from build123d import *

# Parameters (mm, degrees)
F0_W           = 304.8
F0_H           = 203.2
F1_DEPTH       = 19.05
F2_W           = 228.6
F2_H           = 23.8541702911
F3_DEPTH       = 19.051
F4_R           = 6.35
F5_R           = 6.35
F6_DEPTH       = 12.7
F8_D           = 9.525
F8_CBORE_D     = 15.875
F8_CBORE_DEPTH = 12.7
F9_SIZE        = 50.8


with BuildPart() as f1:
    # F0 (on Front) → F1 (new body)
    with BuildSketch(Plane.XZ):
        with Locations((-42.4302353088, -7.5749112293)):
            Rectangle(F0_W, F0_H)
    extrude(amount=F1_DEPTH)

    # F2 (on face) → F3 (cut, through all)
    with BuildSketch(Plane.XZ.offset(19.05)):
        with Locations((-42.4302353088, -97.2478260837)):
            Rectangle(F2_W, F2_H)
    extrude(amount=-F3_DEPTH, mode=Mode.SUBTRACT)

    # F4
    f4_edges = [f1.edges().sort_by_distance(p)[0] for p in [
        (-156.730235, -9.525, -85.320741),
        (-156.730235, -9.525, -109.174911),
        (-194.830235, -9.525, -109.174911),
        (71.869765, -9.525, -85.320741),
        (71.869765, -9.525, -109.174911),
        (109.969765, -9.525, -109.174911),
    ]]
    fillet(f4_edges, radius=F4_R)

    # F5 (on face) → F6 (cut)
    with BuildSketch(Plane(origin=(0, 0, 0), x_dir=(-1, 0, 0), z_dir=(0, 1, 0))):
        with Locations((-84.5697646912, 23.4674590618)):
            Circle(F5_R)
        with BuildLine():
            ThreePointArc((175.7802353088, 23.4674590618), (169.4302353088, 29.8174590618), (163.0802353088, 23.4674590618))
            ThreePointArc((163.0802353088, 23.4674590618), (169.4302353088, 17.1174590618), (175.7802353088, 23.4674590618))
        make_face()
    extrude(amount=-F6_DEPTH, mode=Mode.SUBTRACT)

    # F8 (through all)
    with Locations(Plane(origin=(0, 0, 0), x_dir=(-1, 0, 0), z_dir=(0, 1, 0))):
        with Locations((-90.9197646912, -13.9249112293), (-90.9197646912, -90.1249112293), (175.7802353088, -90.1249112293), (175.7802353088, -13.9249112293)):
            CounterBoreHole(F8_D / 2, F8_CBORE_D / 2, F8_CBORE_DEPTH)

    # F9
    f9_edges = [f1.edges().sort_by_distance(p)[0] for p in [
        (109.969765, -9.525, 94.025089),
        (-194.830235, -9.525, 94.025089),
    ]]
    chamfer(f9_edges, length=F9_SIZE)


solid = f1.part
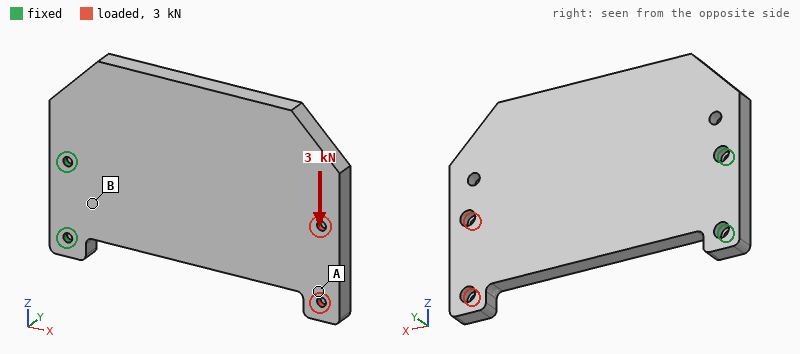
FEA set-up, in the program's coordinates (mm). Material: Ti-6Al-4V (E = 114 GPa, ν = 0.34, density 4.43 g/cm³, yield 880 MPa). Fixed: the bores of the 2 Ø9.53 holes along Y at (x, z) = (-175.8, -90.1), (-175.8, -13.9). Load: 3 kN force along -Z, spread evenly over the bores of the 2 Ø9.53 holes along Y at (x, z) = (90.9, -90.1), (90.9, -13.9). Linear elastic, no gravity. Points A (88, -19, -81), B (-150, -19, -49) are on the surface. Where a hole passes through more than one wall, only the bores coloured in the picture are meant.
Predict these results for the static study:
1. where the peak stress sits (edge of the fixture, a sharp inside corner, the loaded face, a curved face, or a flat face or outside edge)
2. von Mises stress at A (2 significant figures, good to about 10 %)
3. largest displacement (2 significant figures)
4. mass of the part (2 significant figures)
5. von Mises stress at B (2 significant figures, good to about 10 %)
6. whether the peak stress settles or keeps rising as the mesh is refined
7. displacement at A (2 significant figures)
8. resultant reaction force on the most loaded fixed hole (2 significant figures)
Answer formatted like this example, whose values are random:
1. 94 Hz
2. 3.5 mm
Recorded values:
1. edge of the fixture
2. 8.3 MPa
3. 0.18 mm
4. 4.5 kg
5. 17 MPa
6. keeps rising
7. 0.14 mm
8. 10 kN
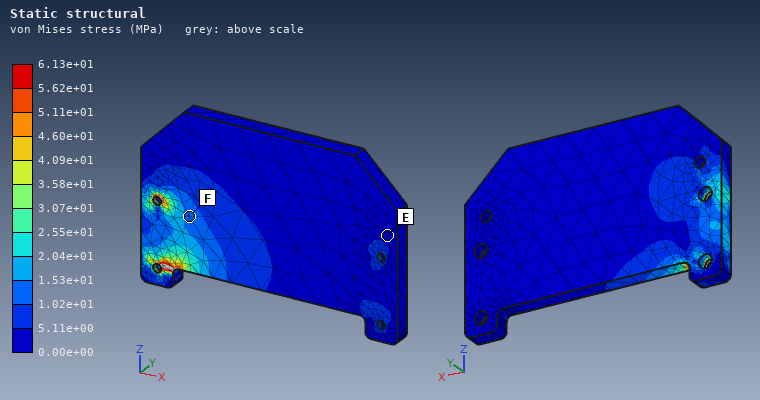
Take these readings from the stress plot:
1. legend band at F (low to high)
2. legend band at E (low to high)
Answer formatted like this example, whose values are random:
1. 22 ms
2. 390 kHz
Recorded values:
1. 1.02e+01 to 1.53e+01 MPa
2. 0.00e+00 to 5.11e+00 MPa
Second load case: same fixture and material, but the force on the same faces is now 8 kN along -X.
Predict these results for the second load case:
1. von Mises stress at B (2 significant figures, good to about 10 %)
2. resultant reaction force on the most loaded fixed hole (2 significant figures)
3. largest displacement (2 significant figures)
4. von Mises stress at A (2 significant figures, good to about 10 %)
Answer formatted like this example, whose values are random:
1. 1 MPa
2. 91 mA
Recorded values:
1. 8.1 MPa
2. 4.1 kN
3. 0.21 mm
4. 24 MPa
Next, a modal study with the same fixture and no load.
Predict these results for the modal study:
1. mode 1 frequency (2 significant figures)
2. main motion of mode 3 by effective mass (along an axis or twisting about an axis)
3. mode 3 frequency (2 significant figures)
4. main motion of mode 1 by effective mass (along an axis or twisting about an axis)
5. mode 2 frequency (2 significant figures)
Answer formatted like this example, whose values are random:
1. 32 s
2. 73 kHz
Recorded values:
1. 110 Hz
2. along Z
3. 610 Hz
4. along Y
5. 460 Hz
